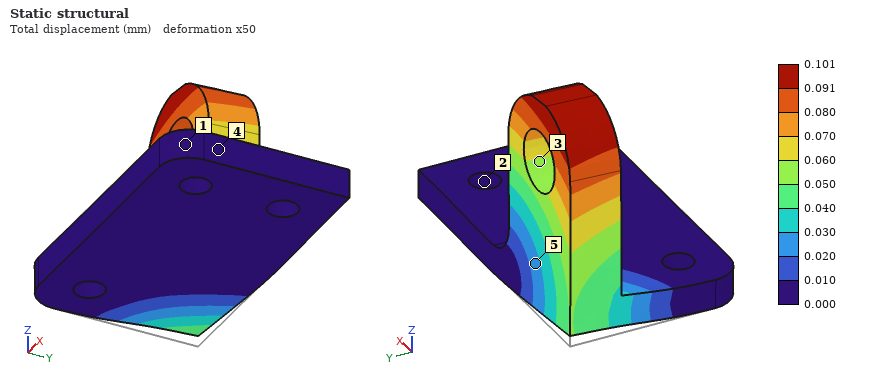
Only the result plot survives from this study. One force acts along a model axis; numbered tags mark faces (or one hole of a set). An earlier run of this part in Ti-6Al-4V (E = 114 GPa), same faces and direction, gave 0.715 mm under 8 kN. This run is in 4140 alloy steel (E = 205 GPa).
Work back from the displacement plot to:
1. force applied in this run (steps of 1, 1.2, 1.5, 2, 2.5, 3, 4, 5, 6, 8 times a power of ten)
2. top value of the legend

2 kN
0.101 mm
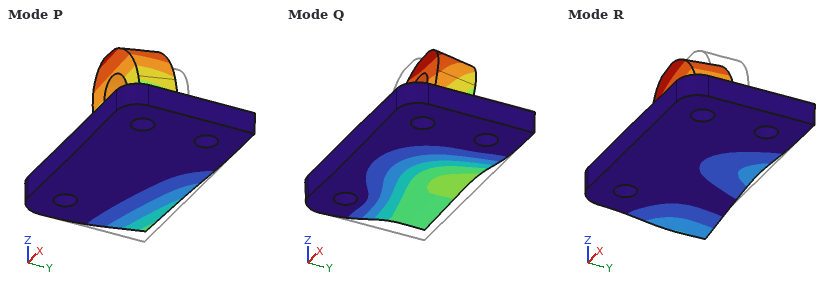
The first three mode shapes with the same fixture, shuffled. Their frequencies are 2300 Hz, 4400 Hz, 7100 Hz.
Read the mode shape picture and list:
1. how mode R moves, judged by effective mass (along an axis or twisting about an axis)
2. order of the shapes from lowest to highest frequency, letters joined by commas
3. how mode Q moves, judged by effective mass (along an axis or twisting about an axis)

along X
P, R, Q
along Z
